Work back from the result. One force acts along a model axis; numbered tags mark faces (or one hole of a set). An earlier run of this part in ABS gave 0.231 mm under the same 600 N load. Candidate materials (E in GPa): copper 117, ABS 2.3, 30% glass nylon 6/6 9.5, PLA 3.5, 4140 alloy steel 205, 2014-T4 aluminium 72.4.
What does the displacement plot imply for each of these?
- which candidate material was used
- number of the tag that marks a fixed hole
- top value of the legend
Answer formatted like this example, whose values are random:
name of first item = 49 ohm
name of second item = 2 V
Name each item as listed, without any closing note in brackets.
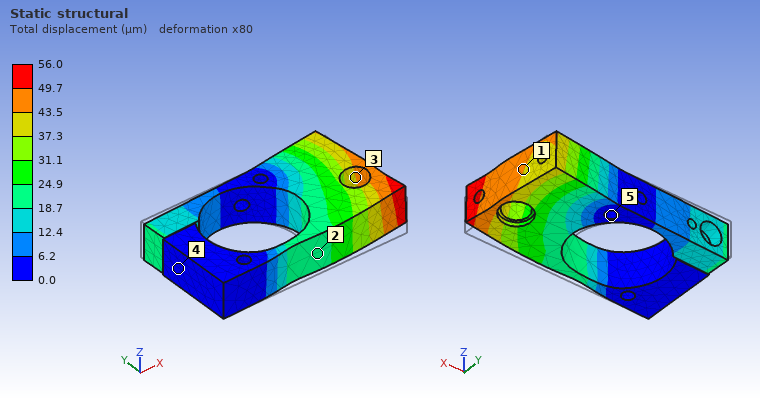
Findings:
which candidate material was used = 30% glass nylon 6/6
number of the tag that marks a fixed hole = 5
top value of the legend = 56.0 µm
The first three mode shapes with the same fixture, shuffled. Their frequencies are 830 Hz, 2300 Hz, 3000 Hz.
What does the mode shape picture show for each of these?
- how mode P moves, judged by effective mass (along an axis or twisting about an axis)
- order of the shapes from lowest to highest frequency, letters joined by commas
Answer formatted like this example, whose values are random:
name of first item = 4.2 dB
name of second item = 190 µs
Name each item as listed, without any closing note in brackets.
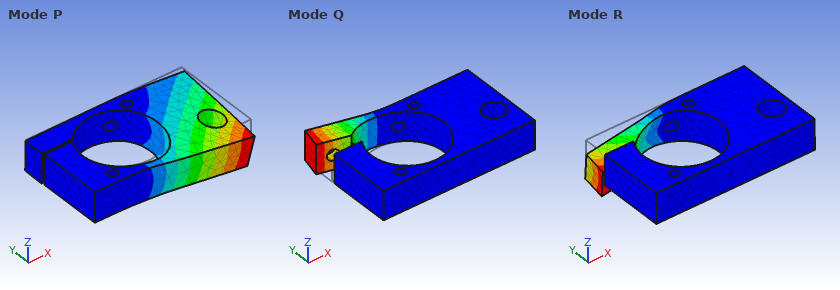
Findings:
how mode P moves, judged by effective mass = along Z
order of the shapes from lowest to highest frequency, letters joined by commas = Q, R, P
